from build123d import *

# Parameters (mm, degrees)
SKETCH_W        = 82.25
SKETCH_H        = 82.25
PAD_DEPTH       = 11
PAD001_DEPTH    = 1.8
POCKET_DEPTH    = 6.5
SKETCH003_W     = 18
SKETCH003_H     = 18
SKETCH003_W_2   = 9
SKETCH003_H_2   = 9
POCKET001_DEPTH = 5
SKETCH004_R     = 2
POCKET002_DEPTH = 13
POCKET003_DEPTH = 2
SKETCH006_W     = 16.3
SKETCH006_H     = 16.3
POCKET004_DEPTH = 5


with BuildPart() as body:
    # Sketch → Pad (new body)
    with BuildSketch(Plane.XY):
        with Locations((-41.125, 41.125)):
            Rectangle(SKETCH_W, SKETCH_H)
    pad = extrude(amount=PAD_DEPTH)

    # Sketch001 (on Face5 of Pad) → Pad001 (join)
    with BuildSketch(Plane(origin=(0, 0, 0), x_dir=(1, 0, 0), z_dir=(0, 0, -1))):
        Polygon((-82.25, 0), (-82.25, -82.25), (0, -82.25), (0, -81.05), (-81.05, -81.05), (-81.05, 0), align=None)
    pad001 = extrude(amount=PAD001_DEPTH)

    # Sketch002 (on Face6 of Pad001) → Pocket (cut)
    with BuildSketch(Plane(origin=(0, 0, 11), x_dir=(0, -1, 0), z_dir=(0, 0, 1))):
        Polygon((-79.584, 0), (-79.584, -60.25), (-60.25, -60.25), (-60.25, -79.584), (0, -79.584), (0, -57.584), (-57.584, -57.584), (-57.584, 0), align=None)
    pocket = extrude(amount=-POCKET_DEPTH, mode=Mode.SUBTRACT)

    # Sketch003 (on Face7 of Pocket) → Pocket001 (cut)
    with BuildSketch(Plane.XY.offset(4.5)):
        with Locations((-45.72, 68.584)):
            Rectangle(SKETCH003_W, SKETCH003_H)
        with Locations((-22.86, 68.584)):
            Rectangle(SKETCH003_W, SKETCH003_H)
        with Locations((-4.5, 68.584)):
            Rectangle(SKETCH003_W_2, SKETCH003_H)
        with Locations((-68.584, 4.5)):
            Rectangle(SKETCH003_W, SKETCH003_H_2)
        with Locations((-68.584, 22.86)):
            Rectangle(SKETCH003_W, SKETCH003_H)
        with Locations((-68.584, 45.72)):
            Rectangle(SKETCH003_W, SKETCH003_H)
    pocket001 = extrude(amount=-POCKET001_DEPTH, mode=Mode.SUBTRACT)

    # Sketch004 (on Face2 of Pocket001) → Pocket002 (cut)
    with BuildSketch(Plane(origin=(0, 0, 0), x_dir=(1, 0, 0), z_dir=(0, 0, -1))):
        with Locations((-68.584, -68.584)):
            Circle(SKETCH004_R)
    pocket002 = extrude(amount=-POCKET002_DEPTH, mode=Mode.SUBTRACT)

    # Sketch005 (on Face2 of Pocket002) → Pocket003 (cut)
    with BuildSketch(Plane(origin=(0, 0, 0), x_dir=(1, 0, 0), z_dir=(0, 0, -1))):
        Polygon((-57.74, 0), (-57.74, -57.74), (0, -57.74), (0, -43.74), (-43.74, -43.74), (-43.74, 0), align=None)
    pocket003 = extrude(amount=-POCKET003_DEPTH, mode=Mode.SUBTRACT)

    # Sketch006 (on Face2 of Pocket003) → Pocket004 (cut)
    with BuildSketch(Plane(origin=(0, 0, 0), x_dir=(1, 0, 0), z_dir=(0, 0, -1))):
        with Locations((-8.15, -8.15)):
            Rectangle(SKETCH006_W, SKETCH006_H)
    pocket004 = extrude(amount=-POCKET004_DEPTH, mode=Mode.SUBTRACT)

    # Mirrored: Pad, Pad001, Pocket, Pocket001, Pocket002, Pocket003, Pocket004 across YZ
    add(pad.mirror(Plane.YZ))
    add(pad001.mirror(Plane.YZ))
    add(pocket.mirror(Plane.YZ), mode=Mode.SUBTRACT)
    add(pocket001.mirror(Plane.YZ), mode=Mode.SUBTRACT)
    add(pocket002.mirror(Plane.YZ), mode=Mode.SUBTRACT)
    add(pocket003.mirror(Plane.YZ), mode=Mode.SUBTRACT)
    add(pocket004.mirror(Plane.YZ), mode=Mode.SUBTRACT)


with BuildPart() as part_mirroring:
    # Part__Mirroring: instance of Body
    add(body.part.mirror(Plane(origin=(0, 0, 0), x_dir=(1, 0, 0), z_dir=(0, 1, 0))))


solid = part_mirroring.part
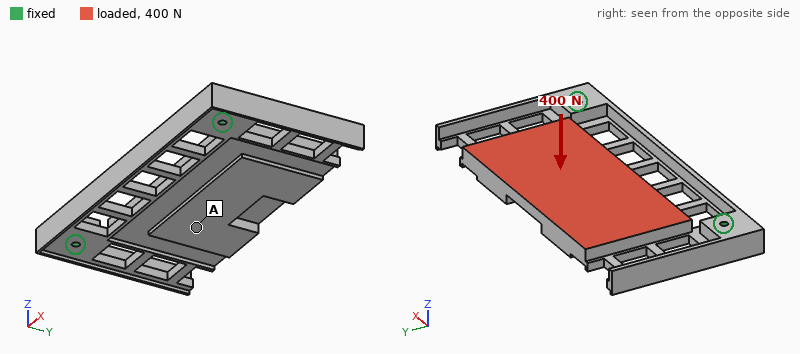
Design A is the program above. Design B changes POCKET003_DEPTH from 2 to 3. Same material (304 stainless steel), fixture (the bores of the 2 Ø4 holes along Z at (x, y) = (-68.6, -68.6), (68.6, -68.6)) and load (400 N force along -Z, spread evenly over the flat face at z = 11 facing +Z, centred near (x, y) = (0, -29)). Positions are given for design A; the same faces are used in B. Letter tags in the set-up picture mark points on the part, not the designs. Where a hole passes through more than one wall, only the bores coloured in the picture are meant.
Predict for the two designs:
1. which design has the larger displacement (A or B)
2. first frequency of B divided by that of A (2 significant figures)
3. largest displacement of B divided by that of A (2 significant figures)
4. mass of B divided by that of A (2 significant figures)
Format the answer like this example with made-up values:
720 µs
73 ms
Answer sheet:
B
0.95
1.1
0.97
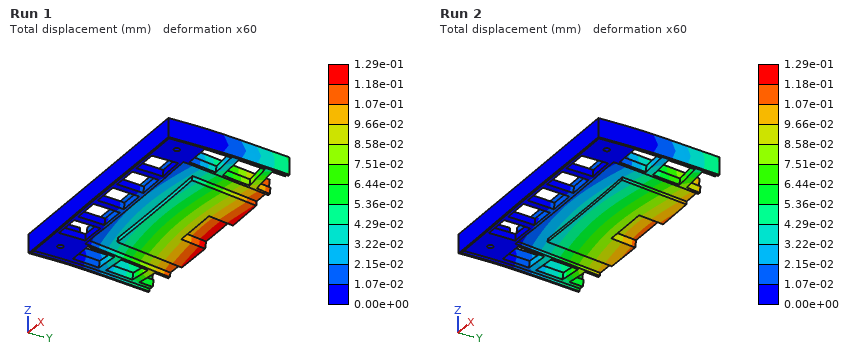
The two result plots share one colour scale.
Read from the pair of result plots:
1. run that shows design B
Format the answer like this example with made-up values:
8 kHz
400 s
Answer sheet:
Run 1
